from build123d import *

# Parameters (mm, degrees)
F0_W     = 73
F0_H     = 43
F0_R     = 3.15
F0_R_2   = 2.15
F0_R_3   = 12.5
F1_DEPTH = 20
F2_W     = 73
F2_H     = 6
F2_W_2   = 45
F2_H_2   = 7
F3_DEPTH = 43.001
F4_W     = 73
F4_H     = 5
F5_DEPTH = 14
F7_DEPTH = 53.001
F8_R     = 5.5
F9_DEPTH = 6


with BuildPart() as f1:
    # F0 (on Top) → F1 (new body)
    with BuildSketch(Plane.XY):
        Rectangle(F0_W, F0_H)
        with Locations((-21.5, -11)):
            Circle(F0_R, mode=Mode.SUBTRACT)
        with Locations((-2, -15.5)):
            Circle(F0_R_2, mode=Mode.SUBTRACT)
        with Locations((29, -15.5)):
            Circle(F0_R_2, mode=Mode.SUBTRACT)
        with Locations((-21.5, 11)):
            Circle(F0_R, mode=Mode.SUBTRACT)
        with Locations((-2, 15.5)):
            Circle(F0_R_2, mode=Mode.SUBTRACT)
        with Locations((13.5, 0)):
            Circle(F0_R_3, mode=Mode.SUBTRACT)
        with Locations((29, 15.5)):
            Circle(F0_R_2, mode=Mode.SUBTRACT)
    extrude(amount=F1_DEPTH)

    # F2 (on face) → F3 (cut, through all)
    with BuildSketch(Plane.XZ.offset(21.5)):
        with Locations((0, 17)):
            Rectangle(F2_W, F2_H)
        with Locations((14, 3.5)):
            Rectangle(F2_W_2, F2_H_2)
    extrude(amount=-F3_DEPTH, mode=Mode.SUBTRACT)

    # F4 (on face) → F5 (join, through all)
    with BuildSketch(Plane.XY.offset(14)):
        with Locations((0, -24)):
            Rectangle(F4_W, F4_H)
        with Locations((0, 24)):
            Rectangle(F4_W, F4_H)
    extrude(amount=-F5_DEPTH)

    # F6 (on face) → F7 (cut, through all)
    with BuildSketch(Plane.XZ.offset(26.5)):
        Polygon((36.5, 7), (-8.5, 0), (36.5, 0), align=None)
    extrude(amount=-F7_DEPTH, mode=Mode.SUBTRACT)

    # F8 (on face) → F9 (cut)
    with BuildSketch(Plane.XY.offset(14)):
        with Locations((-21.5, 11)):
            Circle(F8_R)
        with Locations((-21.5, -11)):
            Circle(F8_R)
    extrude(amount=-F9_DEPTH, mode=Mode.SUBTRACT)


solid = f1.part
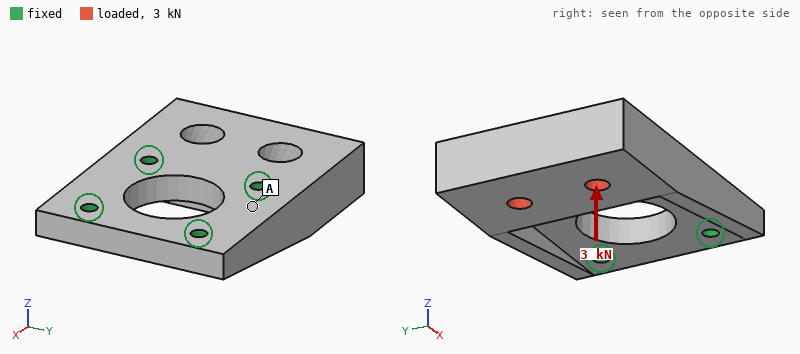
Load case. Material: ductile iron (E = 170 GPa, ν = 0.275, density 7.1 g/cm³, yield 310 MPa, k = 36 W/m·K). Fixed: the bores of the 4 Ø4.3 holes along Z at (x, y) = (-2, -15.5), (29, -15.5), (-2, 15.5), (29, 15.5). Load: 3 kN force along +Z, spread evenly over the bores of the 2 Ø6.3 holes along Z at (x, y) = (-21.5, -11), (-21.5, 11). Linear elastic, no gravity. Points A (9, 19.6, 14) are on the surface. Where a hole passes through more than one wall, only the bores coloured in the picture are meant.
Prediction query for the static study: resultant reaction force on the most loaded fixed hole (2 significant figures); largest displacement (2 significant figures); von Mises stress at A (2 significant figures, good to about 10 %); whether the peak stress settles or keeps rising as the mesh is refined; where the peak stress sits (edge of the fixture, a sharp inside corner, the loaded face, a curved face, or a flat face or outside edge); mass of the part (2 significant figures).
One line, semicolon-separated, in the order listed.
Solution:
2.0 kN; 46 µm; 18 MPa; keeps rising; edge of the fixture; 240 g
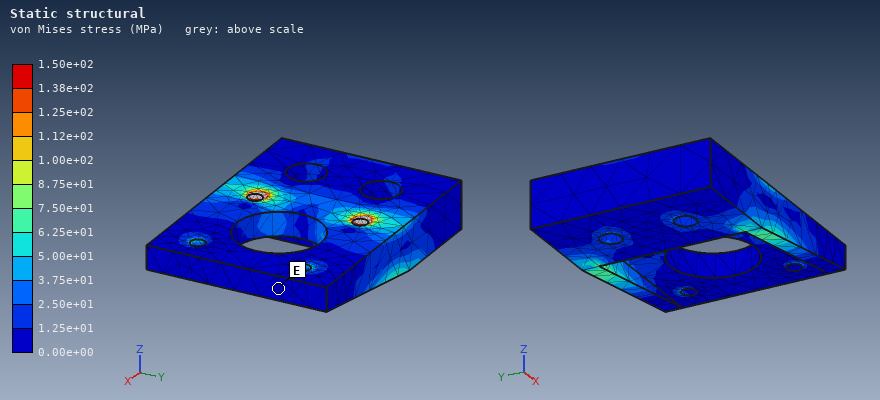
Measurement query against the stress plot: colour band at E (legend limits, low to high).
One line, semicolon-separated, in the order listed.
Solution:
0.00e+00 to 1.25e+01 MPa
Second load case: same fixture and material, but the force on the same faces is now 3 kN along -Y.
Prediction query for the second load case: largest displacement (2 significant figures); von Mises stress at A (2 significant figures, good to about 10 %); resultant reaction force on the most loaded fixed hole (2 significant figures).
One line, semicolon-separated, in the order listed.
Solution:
6.0 µm; 5.5 MPa; 2.1 kN
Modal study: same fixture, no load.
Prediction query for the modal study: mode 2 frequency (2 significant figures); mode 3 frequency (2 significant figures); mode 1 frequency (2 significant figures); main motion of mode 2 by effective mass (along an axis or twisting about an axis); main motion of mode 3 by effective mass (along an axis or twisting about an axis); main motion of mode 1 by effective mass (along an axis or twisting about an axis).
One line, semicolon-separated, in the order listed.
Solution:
8600 Hz; 12 kHz; 4000 Hz; twisting about X; along Y; along Z
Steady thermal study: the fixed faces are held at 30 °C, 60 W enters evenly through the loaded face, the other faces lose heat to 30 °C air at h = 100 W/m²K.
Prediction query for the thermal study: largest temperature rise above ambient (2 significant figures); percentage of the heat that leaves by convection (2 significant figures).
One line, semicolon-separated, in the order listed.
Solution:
67 K; 42 %
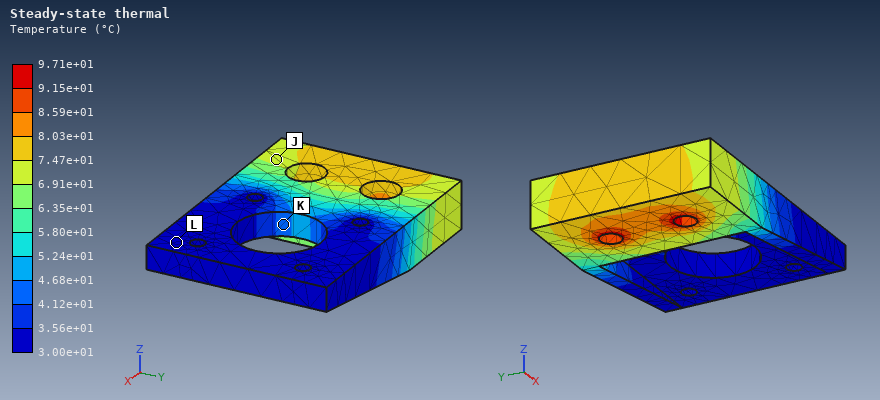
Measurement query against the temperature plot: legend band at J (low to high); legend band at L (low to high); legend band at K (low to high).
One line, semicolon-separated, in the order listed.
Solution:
6.91e+01 to 7.47e+01 °C; 3.00e+01 to 3.56e+01 °C; 4.12e+01 to 4.68e+01 °C
